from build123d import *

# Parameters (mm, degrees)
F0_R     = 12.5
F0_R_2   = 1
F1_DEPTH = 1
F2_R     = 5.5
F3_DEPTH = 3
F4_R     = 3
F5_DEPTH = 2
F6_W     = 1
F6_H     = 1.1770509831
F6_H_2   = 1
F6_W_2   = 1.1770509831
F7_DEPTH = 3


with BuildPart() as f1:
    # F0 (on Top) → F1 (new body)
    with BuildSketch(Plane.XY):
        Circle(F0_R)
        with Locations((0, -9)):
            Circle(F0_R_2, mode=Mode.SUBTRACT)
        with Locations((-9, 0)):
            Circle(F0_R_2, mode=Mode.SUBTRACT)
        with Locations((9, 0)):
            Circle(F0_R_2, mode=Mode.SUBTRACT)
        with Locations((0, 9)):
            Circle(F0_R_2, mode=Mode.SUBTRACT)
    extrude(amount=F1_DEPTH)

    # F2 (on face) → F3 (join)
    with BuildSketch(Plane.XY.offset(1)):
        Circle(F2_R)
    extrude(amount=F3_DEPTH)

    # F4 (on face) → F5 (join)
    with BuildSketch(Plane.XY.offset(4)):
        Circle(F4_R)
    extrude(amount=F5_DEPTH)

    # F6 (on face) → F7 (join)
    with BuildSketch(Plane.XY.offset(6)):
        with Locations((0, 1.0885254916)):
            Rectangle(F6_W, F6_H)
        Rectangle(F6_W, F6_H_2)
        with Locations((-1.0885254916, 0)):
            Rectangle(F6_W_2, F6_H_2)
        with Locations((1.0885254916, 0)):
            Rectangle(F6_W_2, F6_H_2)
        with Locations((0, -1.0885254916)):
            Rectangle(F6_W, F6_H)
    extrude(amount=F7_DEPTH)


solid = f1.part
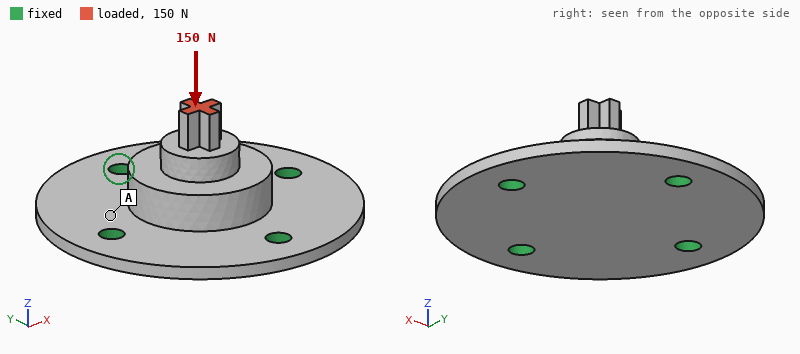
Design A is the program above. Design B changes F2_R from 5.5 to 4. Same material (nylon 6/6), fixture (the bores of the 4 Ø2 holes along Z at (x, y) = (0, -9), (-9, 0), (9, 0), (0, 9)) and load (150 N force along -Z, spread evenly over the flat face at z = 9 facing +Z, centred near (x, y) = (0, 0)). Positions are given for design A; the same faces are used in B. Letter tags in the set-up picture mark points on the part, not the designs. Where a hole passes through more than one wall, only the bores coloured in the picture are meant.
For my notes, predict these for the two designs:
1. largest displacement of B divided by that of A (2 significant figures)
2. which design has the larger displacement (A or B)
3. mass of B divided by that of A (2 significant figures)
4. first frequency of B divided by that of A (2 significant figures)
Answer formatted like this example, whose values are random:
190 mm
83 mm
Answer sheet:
1.9
B
0.84
0.86
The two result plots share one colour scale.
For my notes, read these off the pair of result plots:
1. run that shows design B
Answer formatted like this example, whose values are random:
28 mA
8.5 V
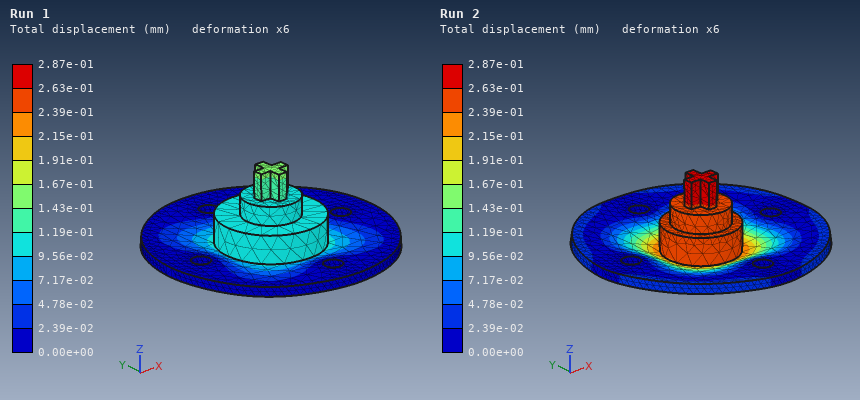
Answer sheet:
Run 2
